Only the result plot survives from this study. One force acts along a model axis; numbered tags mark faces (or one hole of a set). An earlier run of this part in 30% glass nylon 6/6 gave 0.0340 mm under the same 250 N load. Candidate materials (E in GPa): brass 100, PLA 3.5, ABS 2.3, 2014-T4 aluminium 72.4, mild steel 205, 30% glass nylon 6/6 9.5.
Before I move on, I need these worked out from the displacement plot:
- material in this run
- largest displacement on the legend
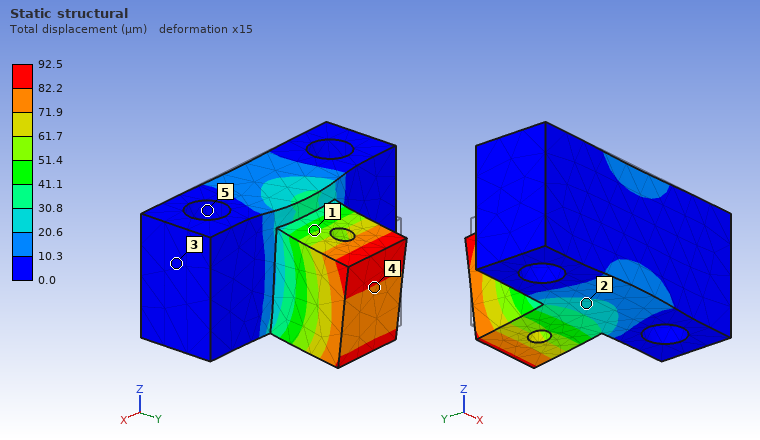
PLA
92.5 µm
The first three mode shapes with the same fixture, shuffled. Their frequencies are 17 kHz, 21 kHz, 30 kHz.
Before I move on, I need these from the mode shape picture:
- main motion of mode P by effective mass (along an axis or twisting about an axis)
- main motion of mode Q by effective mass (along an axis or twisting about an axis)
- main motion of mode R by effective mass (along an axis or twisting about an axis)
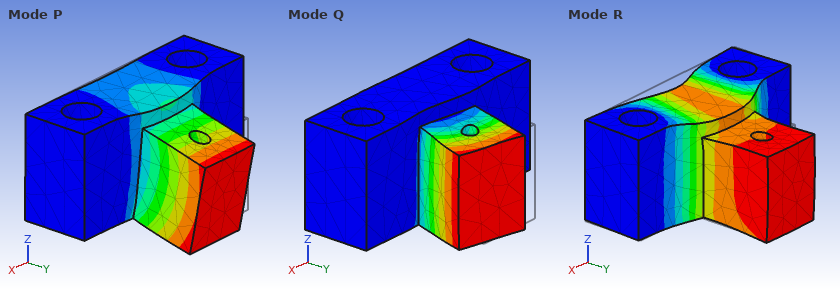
along Z
along X
along Y
